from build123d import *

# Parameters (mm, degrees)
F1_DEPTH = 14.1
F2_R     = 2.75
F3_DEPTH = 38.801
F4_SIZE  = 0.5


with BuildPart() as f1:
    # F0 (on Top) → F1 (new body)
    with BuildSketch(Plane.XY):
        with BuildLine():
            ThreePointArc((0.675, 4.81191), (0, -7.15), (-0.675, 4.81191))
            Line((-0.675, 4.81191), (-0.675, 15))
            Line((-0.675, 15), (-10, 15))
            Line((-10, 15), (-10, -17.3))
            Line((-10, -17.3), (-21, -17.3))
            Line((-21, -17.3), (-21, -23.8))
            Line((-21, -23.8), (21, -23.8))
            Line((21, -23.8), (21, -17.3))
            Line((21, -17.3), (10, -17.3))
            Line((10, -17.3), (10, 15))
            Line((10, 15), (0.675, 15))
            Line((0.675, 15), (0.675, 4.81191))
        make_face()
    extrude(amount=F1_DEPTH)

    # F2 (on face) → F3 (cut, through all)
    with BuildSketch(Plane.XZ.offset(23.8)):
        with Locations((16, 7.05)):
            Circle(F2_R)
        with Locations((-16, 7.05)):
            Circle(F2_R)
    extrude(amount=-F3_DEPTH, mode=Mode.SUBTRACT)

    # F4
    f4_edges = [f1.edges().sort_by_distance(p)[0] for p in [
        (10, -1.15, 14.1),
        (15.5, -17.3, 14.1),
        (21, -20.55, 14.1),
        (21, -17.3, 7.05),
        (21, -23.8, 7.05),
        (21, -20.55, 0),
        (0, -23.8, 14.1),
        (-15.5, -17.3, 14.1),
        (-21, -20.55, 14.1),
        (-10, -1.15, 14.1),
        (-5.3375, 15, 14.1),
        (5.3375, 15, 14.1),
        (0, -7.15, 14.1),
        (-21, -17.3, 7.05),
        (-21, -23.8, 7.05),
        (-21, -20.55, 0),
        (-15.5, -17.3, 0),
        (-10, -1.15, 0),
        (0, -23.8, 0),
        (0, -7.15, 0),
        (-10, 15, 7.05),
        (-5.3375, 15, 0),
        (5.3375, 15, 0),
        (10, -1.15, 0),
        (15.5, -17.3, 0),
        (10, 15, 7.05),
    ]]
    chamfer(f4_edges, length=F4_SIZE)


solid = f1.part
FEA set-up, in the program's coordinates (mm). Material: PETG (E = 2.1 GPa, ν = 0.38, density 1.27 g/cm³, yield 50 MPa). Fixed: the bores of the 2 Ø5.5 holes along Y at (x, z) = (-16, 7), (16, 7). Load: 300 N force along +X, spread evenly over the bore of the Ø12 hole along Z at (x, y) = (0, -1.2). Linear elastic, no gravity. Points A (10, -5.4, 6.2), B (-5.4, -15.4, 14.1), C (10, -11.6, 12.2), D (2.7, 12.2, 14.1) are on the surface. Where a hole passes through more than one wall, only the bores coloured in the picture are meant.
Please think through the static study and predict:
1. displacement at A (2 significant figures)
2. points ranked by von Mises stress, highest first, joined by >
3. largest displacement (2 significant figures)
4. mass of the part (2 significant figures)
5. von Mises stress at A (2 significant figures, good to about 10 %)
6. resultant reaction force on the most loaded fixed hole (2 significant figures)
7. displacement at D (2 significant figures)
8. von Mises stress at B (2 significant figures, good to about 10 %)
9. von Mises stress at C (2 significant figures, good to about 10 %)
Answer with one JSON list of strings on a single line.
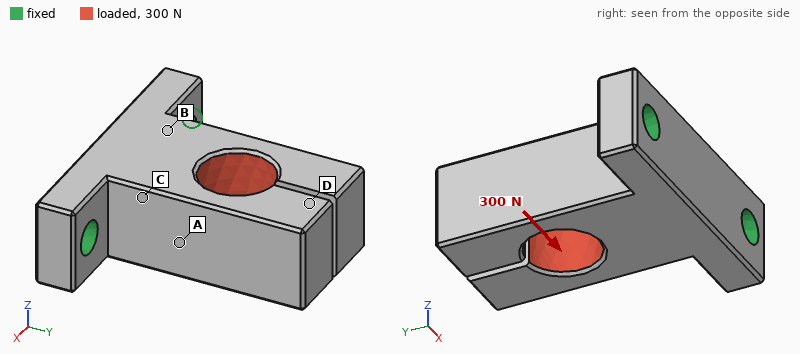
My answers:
["0.11 mm", "A > C > B > D", "0.54 mm", "14 g", "8.5 MPa", "280 N", "0.47 mm", "2.3 MPa", "5.0 MPa"]
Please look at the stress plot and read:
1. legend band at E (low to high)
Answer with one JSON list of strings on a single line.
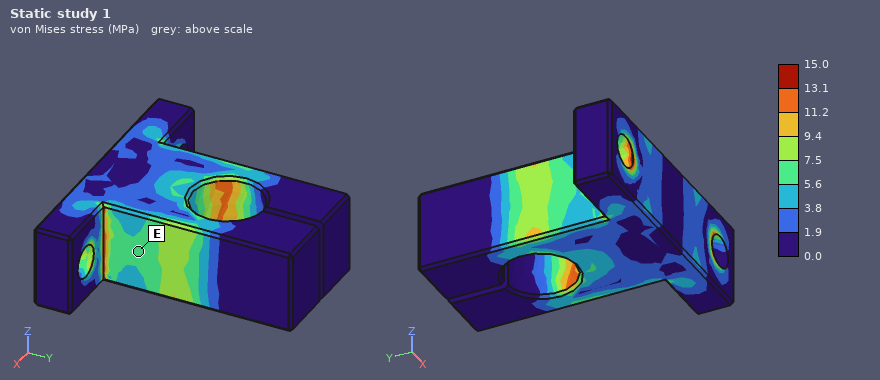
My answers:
["5.6 to 7.5 MPa"]
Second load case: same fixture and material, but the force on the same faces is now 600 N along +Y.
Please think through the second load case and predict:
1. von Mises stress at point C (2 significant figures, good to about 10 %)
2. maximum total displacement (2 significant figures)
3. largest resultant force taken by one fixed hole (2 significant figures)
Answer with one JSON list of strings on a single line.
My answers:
["1.6 MPa", "0.55 mm", "320 N"]
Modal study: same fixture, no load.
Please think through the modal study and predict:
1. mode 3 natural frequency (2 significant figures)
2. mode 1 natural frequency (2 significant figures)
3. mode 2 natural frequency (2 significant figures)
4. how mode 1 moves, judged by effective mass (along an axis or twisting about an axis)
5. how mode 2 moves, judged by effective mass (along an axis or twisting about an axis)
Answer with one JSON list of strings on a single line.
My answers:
["1200 Hz", "1000 Hz", "1200 Hz", "along Z", "along X"]
